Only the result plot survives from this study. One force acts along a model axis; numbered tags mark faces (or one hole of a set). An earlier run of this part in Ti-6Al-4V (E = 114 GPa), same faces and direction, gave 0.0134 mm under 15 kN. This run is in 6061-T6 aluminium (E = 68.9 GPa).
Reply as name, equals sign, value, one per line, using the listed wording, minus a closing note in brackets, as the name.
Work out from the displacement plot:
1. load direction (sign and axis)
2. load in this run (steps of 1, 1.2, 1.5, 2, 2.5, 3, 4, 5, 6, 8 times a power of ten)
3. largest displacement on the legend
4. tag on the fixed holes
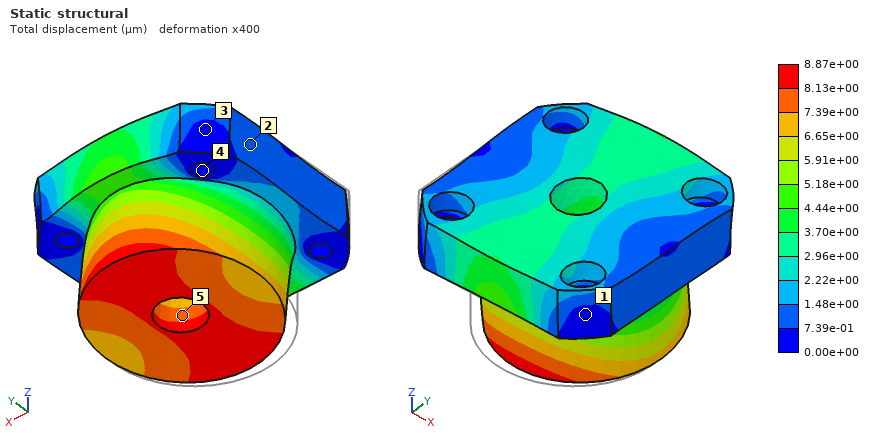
load direction = +Y
load in this run = 6 kN
largest displacement on the legend = 8.87e+00 µm
tag on the fixed holes = 4
